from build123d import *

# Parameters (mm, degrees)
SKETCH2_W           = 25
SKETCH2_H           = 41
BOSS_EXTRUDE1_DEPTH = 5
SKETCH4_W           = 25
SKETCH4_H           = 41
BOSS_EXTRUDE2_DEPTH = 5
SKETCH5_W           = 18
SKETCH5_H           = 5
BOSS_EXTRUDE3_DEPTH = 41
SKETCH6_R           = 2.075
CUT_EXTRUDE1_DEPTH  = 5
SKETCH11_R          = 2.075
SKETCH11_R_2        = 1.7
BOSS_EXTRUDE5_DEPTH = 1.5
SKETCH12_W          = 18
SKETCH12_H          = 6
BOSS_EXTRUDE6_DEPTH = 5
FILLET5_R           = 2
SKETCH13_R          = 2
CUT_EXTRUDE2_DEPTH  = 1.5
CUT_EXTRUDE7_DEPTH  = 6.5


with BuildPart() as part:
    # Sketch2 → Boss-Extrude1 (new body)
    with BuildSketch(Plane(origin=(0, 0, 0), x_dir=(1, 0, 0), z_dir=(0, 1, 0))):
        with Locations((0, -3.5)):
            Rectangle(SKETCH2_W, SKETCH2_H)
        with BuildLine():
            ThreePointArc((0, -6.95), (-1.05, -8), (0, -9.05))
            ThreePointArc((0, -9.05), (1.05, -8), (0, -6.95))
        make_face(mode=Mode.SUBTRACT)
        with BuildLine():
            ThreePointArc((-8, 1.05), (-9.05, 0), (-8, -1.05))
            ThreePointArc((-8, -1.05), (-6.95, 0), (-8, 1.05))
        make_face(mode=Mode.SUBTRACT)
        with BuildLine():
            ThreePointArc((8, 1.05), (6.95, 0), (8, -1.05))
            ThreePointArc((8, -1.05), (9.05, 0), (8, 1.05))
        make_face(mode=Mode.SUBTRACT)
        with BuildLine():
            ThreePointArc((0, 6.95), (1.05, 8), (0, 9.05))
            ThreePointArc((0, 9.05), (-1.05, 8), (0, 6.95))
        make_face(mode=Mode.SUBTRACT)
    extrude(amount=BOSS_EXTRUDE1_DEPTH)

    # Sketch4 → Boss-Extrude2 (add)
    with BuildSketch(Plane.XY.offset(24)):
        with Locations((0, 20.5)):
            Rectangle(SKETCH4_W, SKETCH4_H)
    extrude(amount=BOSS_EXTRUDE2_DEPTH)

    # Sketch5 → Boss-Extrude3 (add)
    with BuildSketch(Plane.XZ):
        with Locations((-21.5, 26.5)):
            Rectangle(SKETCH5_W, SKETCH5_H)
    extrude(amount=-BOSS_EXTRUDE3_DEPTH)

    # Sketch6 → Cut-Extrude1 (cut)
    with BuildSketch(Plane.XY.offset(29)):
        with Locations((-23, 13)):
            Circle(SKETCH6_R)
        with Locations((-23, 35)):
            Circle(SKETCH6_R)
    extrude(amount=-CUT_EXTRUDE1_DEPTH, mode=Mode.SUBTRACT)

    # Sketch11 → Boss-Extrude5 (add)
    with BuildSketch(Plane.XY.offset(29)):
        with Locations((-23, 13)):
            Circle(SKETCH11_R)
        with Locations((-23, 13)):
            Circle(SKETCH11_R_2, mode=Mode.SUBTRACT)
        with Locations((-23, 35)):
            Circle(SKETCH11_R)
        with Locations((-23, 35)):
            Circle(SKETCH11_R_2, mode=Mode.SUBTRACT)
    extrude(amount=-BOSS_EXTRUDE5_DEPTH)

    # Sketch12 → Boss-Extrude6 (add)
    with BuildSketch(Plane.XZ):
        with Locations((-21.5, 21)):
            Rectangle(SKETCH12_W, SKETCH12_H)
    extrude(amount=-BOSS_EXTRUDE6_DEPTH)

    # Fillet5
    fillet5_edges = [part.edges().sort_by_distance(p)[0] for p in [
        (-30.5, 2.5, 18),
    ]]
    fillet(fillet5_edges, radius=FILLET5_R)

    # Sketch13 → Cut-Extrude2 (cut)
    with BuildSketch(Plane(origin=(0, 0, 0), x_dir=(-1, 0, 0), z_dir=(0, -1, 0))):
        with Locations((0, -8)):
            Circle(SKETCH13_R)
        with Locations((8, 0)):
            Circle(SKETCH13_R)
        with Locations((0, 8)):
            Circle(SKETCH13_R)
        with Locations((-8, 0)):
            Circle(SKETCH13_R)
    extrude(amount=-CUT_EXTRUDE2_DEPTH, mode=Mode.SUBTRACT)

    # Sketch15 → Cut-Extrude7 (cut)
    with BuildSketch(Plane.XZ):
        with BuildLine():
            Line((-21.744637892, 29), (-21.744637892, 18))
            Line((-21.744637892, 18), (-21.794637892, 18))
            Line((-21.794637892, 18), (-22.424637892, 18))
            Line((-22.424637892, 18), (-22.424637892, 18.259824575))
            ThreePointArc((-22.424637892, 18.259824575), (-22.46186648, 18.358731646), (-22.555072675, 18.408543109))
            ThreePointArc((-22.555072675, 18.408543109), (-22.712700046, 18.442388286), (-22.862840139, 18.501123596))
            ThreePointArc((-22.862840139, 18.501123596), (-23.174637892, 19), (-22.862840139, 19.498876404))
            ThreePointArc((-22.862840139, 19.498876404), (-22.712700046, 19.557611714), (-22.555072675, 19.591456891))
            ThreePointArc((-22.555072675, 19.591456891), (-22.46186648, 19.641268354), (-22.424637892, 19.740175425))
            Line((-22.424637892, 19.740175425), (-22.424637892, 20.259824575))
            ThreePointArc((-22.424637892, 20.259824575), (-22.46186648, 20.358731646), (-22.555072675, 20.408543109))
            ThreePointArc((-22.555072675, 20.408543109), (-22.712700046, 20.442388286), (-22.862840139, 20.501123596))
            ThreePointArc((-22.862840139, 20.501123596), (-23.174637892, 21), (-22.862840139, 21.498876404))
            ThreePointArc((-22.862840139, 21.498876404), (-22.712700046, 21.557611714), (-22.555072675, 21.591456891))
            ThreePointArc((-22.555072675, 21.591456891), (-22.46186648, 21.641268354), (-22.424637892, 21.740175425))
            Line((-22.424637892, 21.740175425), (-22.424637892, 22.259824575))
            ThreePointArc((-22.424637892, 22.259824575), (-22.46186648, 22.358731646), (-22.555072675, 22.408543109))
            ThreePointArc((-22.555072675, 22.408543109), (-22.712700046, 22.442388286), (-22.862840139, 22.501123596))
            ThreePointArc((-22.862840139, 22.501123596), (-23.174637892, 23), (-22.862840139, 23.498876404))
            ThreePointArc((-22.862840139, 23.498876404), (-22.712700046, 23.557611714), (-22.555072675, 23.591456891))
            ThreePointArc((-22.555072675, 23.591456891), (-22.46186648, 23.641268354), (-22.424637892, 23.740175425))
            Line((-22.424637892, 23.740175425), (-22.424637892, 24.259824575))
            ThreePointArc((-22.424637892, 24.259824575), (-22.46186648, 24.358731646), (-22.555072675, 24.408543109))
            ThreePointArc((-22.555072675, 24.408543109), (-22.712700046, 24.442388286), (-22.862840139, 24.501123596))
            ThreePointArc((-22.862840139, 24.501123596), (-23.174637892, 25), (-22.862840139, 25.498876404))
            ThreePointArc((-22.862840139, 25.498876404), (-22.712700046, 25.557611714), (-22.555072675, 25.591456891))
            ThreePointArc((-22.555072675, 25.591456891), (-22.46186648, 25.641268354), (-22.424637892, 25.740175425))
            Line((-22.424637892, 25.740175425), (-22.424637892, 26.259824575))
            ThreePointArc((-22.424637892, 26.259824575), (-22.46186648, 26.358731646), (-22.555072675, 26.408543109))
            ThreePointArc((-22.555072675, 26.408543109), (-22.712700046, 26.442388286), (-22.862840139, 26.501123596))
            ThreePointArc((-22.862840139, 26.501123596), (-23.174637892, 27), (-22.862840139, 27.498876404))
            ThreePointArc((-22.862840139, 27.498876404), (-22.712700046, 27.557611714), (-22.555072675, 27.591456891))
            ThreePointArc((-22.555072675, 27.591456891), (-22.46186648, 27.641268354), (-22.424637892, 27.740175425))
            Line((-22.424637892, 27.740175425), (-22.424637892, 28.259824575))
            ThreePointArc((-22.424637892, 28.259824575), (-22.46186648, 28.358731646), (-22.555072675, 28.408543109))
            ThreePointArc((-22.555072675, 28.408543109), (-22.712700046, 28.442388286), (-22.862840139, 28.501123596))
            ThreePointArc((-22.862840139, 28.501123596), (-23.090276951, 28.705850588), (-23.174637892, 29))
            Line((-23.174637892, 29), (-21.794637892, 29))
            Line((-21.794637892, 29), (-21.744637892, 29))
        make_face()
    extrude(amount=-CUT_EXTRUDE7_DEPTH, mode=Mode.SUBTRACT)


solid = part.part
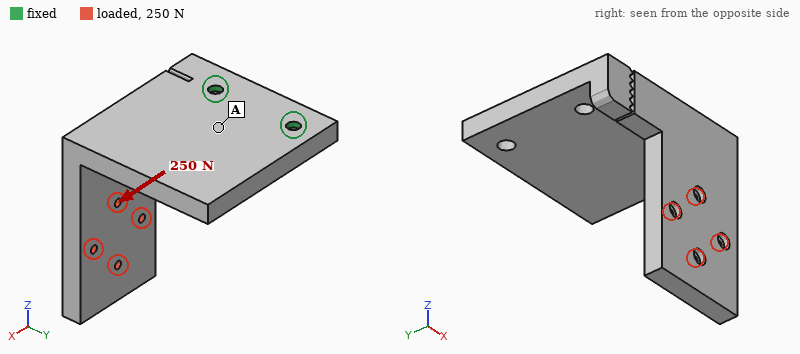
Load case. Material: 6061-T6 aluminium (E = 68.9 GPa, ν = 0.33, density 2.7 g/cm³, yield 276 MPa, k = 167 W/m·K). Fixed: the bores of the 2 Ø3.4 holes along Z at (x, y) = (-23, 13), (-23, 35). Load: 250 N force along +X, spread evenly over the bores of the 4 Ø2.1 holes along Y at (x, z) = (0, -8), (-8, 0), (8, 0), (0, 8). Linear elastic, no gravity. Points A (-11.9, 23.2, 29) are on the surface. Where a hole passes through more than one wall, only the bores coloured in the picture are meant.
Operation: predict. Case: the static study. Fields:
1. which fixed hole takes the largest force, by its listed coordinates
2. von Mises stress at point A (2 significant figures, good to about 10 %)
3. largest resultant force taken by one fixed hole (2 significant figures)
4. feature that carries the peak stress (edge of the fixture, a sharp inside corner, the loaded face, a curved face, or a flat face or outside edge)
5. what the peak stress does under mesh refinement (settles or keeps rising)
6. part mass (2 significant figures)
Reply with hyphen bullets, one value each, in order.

- (-23, 13)
- 31 MPa
- 370 N
- edge of the fixture
- keeps rising
- 38 g
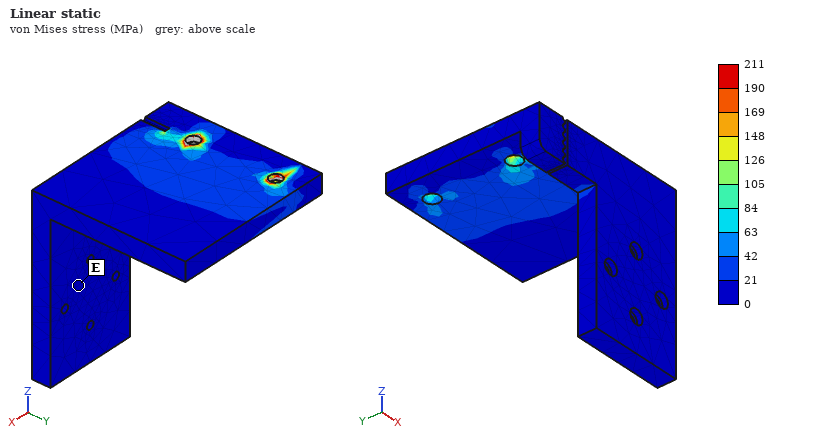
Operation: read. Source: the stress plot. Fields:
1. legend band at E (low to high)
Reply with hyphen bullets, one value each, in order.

- 0 to 21 MPa
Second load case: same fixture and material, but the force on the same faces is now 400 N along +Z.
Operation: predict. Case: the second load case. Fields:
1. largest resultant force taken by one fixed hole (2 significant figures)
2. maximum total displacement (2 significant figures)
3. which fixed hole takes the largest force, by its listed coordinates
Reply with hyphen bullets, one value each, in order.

- 550 N
- 0.62 mm
- (-23, 13)
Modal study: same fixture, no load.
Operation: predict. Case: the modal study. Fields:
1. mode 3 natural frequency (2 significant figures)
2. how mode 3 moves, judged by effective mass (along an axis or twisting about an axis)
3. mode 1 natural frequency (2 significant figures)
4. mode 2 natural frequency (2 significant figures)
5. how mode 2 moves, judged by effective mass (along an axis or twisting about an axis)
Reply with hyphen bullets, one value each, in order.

- 4600 Hz
- along Z
- 940 Hz
- 1500 Hz
- along Y
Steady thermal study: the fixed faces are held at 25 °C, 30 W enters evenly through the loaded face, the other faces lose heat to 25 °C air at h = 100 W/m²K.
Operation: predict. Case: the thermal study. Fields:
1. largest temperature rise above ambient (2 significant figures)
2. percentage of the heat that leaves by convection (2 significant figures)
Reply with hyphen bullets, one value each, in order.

- 47 K
- 46 %
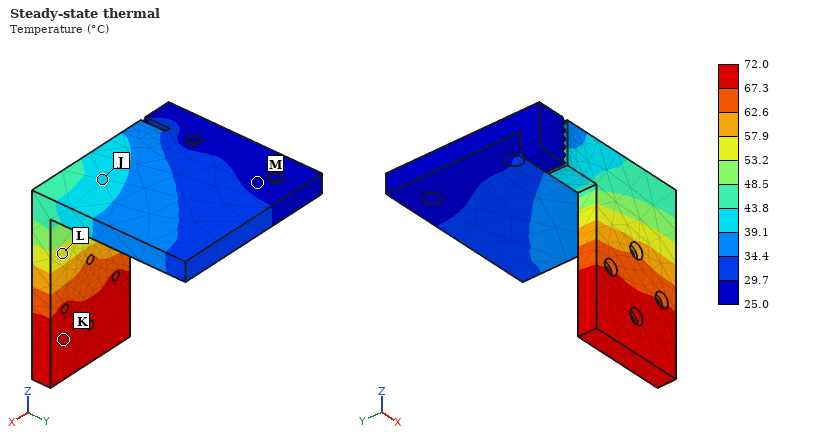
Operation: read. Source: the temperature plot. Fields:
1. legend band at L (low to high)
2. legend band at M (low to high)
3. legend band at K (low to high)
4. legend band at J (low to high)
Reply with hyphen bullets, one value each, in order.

- 53.2 to 57.9 °C
- 25.0 to 29.7 °C
- 67.3 to 72.0 °C
- 39.1 to 43.8 °C
